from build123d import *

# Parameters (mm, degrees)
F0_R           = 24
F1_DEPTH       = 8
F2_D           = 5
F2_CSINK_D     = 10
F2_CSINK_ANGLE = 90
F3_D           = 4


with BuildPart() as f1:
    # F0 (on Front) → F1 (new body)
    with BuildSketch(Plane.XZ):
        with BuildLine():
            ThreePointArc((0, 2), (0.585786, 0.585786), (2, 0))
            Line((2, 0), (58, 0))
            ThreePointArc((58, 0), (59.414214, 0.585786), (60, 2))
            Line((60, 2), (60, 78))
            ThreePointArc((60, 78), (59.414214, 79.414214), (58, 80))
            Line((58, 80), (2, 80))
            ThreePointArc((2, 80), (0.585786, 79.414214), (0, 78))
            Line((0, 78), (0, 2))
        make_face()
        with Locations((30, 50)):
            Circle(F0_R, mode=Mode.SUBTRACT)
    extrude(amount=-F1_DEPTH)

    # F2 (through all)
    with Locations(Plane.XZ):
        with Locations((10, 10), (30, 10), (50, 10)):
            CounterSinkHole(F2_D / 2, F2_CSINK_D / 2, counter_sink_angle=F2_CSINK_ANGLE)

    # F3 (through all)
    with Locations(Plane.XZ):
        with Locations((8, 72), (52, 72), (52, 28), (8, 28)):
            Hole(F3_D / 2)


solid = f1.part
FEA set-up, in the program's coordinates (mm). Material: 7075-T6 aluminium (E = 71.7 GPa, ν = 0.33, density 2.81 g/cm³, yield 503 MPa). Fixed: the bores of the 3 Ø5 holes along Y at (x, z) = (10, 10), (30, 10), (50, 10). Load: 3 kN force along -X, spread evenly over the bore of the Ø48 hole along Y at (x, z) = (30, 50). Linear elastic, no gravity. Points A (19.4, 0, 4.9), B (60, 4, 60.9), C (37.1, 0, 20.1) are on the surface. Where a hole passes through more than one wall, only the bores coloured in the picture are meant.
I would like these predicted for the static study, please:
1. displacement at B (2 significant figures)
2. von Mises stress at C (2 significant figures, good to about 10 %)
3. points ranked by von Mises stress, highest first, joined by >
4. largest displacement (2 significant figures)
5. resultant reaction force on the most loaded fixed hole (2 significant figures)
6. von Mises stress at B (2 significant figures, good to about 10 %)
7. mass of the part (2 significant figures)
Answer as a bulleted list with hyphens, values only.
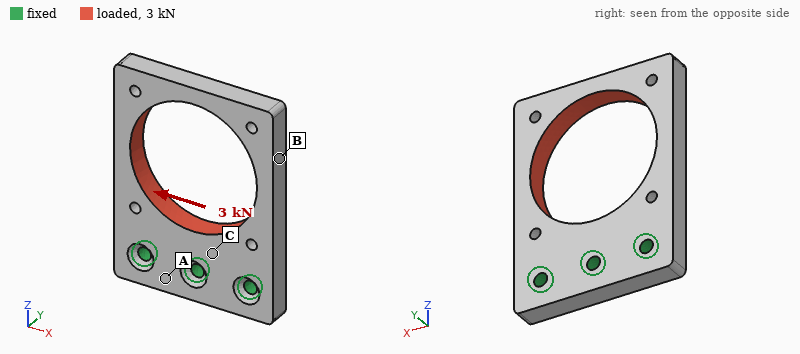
- 0.18 mm
- 29 MPa
- B > C > A
- 0.22 mm
- 2.8 kN
- 69 MPa
- 64 g
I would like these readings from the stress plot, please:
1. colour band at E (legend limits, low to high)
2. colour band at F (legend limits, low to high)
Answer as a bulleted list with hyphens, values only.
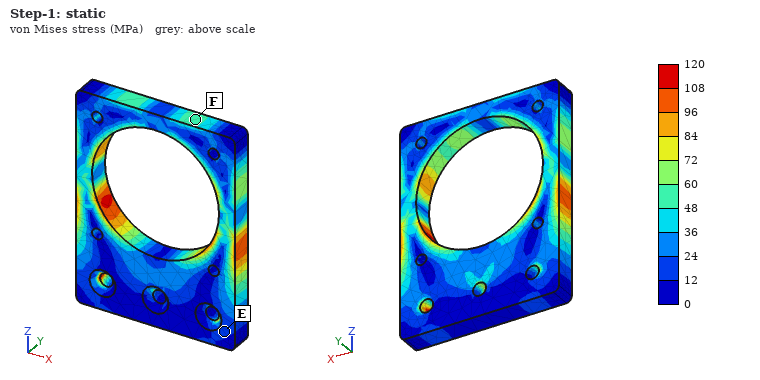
- 12 to 24 MPa
- 48 to 60 MPa
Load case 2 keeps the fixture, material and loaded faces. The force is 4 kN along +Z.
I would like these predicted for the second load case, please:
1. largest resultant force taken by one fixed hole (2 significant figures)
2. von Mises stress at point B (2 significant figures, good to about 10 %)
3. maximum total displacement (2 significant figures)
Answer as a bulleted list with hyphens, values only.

- 2.0 kN
- 22 MPa
- 64 µm
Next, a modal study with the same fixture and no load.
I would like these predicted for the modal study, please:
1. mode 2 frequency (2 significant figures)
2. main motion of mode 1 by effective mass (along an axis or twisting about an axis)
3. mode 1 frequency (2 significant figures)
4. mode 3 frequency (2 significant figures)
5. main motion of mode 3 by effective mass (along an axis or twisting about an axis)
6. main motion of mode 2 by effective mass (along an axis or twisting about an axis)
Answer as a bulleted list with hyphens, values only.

- 2400 Hz
- along Y
- 1100 Hz
- 3200 Hz
- along X
- twisting about Z
